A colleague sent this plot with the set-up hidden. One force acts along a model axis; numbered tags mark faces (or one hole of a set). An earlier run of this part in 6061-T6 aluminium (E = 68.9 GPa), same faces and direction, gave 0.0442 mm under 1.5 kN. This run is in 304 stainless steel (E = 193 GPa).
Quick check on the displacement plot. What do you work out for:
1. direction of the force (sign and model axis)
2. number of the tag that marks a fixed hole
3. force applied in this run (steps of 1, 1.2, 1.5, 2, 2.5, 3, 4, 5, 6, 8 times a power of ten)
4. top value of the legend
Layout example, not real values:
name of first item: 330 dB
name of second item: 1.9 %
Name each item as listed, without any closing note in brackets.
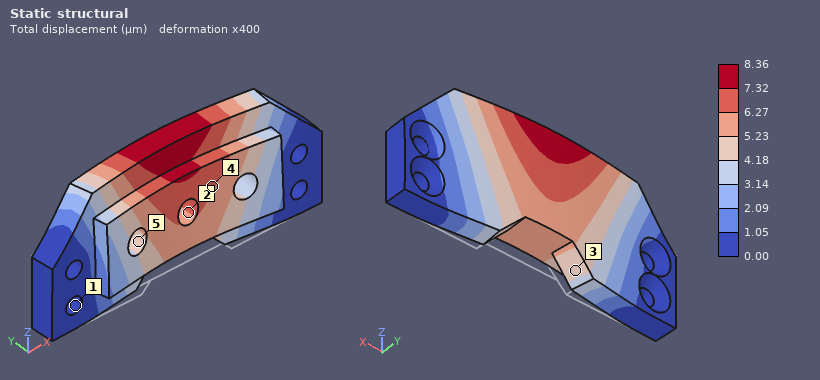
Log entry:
direction of the force: +Y
number of the tag that marks a fixed hole: 1
force applied in this run: 800 N
top value of the legend: 8.36 µm
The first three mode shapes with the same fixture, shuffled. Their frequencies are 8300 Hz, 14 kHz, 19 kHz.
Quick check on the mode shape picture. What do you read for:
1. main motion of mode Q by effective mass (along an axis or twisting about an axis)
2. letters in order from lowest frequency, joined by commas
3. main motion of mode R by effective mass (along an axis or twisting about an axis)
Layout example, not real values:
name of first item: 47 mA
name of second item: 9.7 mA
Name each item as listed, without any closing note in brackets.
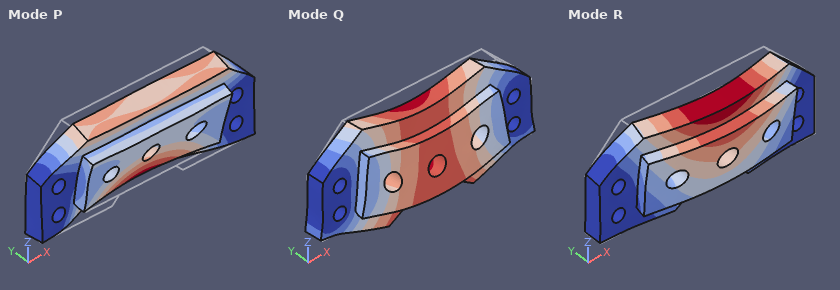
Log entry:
main motion of mode Q by effective mass: along Z
letters in order from lowest frequency, joined by commas: R, P, Q
main motion of mode R by effective mass: along Y
